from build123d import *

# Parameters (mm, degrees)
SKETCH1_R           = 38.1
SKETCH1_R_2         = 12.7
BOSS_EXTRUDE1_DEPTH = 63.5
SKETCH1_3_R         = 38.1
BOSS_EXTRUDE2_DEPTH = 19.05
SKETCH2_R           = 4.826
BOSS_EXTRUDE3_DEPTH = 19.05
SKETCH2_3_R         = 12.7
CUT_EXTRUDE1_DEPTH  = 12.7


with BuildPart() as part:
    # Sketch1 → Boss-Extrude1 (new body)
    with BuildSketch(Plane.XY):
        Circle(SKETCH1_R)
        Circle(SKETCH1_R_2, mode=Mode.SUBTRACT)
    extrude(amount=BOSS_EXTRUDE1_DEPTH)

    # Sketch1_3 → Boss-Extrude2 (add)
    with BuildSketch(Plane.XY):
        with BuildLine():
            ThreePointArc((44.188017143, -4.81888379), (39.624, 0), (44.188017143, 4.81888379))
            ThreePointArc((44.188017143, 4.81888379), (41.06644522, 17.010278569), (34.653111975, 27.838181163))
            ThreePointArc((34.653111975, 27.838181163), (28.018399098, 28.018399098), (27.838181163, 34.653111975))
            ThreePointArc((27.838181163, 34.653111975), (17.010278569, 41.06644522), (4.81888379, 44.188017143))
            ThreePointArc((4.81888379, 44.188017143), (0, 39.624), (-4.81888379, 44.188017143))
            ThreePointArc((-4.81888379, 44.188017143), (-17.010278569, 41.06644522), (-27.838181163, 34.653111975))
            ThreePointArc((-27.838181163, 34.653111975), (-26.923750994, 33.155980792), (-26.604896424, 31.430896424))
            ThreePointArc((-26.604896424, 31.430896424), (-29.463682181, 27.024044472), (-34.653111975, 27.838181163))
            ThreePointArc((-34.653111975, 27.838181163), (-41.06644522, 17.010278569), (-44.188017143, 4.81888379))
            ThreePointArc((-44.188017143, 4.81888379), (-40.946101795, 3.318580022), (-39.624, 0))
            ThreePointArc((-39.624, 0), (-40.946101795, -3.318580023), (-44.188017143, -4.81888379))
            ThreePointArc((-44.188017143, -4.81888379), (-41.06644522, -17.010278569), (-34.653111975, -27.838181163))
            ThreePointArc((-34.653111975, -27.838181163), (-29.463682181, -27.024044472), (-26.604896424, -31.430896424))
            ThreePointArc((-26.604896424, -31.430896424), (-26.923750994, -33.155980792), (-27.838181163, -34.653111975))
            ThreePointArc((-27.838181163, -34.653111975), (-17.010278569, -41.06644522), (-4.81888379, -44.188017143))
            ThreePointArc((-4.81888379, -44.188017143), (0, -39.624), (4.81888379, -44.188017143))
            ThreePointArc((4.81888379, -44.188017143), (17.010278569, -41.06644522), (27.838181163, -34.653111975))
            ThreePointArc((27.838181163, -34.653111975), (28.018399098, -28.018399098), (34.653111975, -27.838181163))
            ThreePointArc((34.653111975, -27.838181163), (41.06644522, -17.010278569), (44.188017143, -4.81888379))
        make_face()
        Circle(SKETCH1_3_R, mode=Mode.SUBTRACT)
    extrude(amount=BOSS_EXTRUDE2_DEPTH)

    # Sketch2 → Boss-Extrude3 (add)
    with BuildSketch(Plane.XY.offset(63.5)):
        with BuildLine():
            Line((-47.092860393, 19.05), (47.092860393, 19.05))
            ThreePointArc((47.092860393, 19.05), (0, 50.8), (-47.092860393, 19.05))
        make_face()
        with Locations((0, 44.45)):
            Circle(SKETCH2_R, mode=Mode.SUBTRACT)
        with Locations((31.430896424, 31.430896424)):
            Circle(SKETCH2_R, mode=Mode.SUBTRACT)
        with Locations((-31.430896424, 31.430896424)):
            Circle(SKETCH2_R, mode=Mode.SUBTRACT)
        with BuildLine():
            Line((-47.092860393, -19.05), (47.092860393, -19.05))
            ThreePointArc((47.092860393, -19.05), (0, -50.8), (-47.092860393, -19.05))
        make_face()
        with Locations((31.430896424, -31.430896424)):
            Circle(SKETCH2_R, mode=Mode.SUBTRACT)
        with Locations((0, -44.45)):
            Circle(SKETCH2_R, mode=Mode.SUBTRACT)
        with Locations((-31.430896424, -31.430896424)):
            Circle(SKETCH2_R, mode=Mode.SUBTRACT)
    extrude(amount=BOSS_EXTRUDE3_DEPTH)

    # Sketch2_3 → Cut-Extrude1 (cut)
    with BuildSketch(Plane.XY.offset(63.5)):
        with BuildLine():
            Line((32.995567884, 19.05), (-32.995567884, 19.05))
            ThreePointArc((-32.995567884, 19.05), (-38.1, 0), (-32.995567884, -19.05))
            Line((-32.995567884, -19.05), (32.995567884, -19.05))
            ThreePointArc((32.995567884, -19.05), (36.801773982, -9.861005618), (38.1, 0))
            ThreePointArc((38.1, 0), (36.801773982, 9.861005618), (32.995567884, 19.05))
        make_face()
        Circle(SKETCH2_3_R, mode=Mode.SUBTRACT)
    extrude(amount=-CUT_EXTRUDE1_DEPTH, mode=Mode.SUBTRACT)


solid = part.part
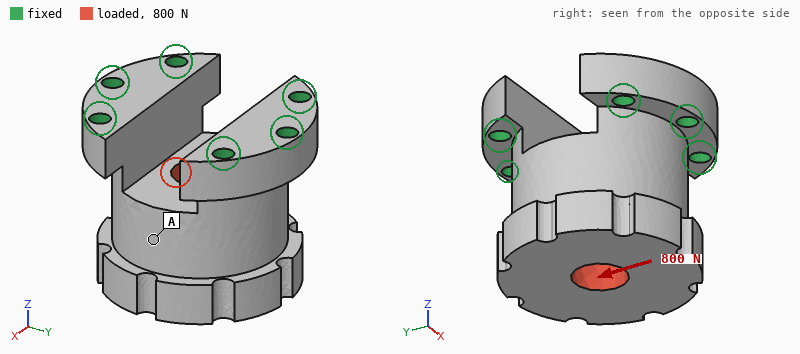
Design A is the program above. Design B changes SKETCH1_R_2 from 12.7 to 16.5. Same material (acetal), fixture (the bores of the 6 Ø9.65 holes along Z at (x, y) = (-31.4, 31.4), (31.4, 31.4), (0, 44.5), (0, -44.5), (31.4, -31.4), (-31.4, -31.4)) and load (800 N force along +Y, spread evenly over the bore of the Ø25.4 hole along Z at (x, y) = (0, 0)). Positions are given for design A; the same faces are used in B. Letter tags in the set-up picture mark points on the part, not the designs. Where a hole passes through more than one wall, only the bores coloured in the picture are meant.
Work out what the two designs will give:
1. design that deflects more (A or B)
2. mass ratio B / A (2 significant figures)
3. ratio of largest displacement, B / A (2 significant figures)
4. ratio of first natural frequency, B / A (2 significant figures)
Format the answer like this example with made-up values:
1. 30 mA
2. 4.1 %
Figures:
1. B
2. 0.95
3. 1.1
4. 1.0
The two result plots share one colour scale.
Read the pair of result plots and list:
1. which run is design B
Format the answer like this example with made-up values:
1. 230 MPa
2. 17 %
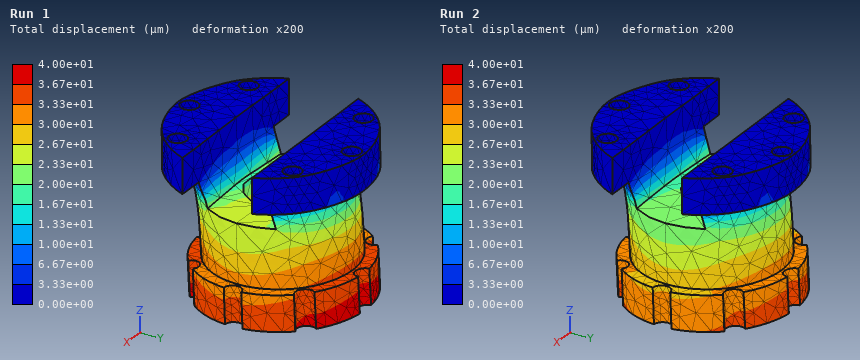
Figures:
1. Run 1
